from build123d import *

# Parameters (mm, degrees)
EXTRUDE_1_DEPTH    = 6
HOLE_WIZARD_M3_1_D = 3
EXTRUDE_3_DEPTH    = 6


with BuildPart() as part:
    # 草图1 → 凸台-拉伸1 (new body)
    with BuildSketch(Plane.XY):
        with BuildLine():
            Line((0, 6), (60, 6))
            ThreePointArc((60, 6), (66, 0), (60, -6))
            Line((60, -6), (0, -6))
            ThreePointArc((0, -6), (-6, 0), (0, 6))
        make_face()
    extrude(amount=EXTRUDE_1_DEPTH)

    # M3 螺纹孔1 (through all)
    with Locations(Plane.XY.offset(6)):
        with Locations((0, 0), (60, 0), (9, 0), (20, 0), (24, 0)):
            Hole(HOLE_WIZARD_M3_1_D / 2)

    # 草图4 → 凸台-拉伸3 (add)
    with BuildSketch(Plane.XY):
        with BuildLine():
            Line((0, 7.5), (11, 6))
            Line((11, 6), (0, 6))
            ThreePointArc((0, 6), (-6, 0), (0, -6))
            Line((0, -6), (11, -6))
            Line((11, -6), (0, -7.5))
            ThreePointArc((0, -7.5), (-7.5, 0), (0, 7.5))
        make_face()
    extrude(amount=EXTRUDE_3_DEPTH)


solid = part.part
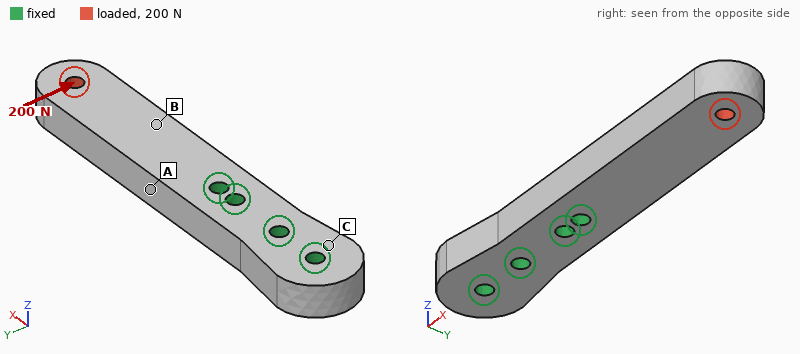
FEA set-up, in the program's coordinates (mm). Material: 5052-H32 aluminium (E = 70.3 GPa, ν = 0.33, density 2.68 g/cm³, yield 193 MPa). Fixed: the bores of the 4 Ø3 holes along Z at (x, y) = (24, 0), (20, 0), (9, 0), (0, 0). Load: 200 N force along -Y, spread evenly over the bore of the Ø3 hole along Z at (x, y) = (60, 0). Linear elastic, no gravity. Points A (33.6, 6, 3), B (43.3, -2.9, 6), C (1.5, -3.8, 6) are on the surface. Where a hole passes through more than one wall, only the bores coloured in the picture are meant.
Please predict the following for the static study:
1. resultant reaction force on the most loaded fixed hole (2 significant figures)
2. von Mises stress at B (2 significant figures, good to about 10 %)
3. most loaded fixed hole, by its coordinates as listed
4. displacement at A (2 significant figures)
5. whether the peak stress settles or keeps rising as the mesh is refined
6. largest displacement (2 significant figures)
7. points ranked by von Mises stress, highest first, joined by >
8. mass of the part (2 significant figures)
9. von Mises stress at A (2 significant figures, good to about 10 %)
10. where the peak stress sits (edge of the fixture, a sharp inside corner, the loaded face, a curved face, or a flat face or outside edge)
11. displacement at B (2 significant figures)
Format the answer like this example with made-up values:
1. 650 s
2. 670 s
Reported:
1. 750 N
2. 13 MPa
3. (24, 0)
4. 14 µm
5. keeps rising
6. 89 µm
7. A > B > C
8. 14 g
9. 37 MPa
10. edge of the fixture
11. 30 µm
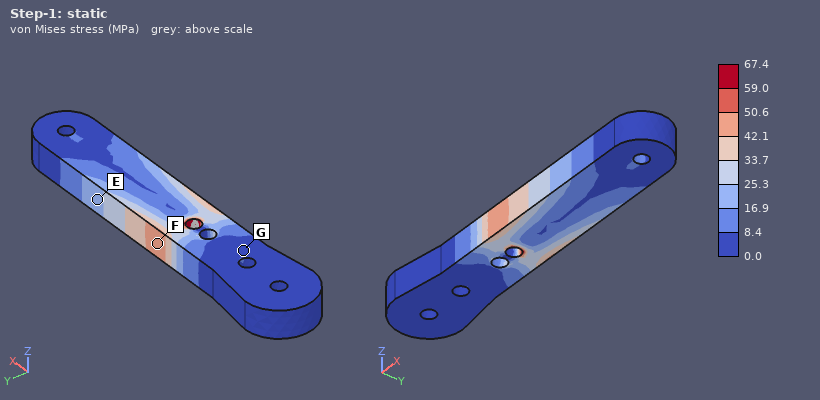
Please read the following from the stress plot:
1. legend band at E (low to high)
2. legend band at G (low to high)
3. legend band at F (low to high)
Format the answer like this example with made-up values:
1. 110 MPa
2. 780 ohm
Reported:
1. 16.9 to 25.3 MPa
2. 0.0 to 8.4 MPa
3. 42.1 to 50.6 MPa
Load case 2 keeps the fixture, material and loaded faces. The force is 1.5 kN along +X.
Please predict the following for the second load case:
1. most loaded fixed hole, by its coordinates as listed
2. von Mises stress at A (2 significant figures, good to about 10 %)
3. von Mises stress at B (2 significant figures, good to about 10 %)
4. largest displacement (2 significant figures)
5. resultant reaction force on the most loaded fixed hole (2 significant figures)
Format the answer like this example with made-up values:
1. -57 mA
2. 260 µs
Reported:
1. (24, 0)
2. 20 MPa
3. 21 MPa
4. 13 µm
5. 1.1 kN
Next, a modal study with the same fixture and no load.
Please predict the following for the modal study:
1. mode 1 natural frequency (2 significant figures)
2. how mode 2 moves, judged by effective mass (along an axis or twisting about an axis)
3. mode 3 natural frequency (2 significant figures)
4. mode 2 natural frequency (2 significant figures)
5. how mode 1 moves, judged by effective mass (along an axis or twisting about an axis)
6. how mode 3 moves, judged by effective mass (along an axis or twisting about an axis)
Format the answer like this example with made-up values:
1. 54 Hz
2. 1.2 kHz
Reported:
1. 3000 Hz
2. along Y
3. 15 kHz
4. 4900 Hz
5. along Z
6. twisting about X
